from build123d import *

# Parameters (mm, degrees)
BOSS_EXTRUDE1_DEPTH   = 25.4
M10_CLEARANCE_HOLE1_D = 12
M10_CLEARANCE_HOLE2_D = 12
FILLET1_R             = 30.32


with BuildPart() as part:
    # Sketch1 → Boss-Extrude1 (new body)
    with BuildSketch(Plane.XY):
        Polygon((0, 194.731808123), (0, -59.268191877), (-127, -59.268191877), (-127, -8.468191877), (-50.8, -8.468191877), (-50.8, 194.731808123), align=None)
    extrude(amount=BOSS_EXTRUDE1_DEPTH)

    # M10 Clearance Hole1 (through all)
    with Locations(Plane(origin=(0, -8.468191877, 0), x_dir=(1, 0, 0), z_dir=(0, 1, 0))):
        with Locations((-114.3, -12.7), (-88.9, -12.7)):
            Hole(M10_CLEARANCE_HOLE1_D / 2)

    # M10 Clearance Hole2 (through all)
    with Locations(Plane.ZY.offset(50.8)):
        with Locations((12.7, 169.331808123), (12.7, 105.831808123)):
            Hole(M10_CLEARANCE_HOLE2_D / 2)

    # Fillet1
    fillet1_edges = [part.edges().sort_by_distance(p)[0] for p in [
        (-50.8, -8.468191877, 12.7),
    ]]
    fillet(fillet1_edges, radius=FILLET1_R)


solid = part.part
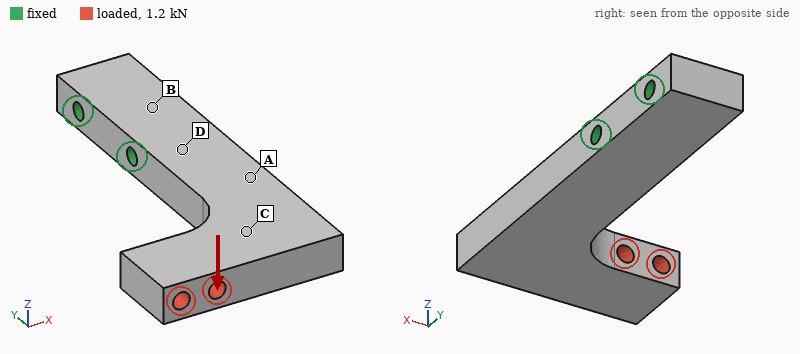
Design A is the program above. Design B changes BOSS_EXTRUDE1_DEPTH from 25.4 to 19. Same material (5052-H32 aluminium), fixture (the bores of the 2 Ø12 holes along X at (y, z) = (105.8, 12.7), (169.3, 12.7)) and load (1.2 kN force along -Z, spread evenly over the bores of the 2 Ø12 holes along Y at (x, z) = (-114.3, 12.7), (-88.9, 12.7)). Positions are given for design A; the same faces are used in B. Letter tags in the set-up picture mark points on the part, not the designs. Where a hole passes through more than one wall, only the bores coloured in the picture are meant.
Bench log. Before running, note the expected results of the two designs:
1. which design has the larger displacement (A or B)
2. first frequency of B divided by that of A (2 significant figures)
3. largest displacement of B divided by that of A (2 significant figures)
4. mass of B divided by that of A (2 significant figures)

B
0.80
2.2
0.73
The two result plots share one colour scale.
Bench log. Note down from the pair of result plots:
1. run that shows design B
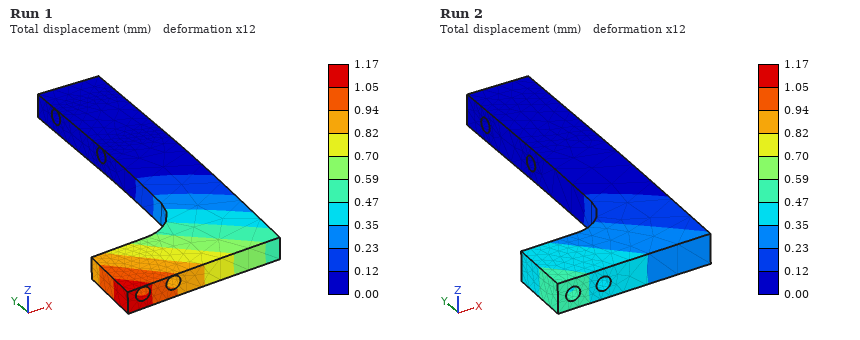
Run 1
